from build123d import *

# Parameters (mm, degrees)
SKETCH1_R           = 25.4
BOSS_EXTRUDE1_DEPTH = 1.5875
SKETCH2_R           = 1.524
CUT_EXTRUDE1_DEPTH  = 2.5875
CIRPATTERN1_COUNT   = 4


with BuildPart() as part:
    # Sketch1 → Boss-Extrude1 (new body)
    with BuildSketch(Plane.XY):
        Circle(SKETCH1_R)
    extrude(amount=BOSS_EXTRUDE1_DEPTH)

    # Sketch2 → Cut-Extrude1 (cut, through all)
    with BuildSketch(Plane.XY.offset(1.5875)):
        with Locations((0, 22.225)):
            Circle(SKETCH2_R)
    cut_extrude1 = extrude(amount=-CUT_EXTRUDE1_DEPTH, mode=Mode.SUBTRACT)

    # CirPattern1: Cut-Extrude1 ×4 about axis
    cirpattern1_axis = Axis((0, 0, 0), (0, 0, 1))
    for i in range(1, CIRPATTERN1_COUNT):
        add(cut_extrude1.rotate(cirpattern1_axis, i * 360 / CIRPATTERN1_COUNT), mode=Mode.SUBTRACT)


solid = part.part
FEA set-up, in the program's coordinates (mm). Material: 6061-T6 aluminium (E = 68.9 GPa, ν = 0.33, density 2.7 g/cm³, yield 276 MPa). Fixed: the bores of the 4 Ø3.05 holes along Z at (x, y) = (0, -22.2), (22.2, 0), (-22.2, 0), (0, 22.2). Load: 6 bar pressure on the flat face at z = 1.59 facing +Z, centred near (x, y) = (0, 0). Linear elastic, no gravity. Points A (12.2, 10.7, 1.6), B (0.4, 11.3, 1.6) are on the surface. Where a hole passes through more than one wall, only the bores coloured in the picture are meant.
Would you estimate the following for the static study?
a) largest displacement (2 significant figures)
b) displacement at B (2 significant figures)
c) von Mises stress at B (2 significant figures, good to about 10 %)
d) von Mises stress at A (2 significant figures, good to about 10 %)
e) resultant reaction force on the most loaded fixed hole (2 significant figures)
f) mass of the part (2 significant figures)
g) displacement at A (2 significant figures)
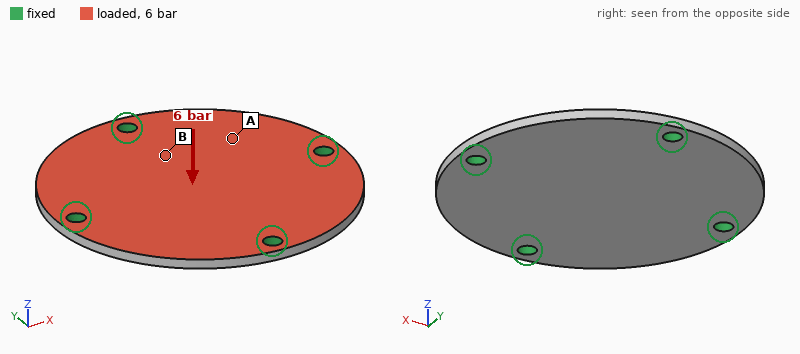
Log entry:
0.13 mm
0.082 mm
33 MPa
67 MPa
300 N
8.6 g
0.078 mm
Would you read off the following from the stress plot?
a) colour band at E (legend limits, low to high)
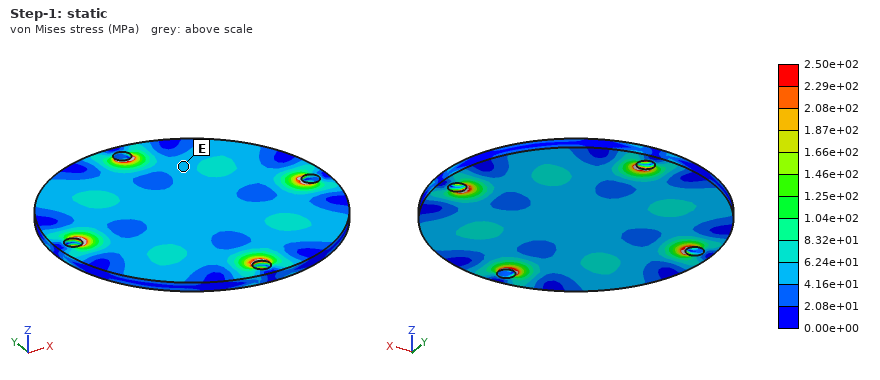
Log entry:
4.16e+01 to 6.24e+01 MPa
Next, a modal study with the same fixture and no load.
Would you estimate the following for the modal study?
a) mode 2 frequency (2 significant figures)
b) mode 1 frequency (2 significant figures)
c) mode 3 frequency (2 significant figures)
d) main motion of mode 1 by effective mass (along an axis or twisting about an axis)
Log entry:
7500 Hz
6300 Hz
7800 Hz
along Z
